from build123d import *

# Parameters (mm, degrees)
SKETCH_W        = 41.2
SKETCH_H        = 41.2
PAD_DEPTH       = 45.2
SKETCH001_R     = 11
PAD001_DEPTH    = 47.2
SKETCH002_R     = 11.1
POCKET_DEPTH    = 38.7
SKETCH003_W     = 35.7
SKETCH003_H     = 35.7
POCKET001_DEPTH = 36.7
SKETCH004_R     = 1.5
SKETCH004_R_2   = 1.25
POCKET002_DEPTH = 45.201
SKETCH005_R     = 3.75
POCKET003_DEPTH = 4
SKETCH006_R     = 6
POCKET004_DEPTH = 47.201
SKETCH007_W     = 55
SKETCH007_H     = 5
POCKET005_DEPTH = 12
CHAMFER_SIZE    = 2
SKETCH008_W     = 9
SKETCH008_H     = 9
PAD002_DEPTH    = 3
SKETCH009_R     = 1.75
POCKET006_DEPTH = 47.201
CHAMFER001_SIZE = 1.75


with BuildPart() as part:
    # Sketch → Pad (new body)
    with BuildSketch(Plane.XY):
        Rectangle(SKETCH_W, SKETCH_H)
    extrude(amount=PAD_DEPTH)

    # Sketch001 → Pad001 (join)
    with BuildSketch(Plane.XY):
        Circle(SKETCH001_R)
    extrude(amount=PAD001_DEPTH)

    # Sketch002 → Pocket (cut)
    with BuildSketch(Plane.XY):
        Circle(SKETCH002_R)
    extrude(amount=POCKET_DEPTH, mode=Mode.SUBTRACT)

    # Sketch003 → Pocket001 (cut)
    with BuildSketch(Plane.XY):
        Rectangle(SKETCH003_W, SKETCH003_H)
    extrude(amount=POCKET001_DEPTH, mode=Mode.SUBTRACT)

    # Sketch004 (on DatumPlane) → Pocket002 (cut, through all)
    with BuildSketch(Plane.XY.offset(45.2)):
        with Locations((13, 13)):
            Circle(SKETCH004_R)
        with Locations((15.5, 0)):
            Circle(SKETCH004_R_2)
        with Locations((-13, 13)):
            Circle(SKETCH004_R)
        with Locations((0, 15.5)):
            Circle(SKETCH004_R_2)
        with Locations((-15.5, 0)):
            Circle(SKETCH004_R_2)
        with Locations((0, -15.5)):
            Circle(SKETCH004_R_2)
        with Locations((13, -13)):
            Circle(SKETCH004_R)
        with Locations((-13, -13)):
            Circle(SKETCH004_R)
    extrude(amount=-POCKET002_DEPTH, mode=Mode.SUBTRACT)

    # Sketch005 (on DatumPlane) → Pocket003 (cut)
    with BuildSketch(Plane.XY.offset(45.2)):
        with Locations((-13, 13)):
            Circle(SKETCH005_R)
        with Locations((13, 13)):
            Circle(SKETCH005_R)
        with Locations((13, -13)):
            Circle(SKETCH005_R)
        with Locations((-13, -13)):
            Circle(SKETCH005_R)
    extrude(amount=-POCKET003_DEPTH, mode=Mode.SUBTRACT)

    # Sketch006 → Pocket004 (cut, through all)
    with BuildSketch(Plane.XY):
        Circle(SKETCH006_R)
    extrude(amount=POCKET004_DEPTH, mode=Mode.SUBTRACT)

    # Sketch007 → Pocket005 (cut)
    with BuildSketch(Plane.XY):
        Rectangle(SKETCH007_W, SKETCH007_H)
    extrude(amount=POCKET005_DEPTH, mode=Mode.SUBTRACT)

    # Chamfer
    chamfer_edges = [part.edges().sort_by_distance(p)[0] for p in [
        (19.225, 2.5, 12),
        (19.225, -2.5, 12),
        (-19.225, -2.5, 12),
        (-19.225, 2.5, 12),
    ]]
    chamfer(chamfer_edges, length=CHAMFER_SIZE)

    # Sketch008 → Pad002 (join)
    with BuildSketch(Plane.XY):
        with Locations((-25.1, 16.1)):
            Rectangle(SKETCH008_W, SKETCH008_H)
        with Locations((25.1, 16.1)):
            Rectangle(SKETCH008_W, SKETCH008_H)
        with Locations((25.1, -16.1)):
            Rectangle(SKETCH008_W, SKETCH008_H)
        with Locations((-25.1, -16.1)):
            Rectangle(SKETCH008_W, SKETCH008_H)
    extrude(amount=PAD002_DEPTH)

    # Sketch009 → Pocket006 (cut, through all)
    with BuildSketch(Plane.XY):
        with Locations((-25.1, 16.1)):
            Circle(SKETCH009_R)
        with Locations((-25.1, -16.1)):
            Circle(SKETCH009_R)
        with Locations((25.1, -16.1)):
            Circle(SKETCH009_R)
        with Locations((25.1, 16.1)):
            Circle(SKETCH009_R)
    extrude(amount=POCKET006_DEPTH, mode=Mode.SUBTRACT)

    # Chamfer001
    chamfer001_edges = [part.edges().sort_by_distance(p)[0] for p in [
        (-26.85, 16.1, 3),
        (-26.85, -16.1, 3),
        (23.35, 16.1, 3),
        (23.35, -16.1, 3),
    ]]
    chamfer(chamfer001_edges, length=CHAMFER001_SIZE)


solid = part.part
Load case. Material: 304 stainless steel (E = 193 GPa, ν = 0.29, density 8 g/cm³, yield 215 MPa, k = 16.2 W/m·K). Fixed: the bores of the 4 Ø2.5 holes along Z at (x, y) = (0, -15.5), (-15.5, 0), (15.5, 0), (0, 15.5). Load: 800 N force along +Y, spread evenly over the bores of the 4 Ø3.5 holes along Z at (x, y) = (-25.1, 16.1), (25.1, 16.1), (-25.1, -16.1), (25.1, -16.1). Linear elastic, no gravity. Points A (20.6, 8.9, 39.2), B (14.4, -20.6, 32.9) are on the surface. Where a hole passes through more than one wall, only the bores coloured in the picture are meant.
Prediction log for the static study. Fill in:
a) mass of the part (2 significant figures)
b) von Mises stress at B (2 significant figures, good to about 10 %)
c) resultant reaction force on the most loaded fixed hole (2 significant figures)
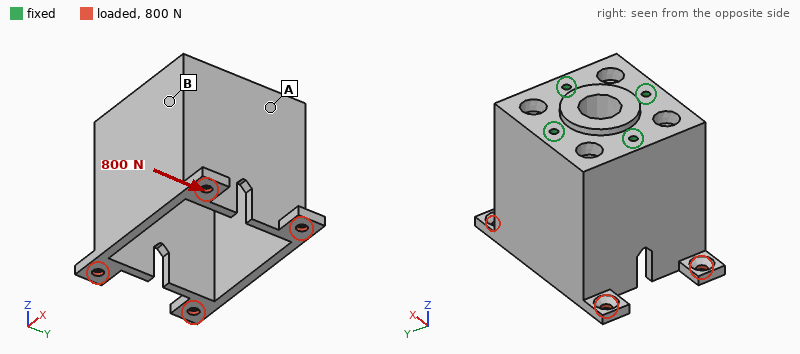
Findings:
230 g
8.1 MPa
790 N
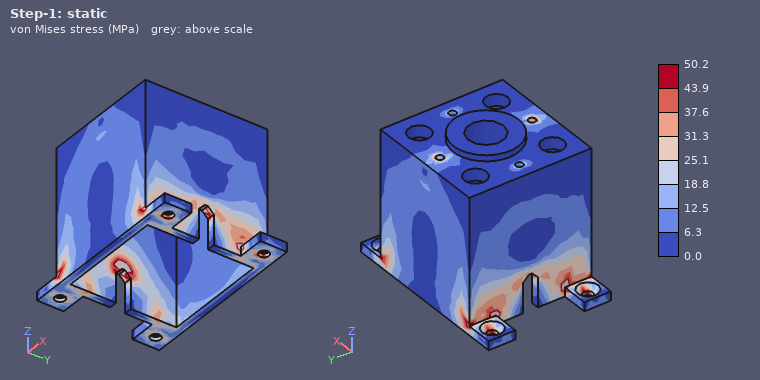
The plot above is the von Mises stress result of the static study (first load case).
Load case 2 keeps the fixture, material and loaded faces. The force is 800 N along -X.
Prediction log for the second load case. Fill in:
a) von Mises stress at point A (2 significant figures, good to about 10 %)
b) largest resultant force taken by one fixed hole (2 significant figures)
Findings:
9.2 MPa
780 N
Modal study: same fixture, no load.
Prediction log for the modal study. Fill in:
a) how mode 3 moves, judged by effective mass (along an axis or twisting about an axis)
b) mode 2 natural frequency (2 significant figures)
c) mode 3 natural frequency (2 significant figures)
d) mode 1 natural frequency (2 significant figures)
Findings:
along X
5000 Hz
5800 Hz
4600 Hz
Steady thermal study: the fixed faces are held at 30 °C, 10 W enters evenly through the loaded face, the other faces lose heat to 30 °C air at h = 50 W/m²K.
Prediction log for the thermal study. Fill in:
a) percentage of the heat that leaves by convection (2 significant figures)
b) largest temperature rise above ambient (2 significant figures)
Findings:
83 %
72 K
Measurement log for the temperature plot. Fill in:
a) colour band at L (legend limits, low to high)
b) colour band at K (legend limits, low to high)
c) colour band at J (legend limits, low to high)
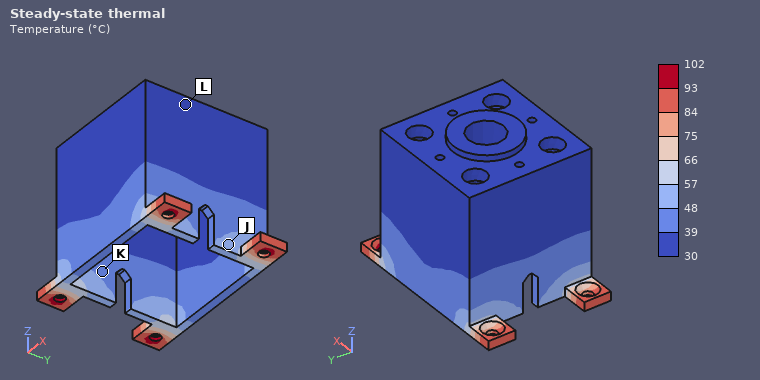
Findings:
30 to 39 °C
39 to 48 °C
48 to 57 °C
